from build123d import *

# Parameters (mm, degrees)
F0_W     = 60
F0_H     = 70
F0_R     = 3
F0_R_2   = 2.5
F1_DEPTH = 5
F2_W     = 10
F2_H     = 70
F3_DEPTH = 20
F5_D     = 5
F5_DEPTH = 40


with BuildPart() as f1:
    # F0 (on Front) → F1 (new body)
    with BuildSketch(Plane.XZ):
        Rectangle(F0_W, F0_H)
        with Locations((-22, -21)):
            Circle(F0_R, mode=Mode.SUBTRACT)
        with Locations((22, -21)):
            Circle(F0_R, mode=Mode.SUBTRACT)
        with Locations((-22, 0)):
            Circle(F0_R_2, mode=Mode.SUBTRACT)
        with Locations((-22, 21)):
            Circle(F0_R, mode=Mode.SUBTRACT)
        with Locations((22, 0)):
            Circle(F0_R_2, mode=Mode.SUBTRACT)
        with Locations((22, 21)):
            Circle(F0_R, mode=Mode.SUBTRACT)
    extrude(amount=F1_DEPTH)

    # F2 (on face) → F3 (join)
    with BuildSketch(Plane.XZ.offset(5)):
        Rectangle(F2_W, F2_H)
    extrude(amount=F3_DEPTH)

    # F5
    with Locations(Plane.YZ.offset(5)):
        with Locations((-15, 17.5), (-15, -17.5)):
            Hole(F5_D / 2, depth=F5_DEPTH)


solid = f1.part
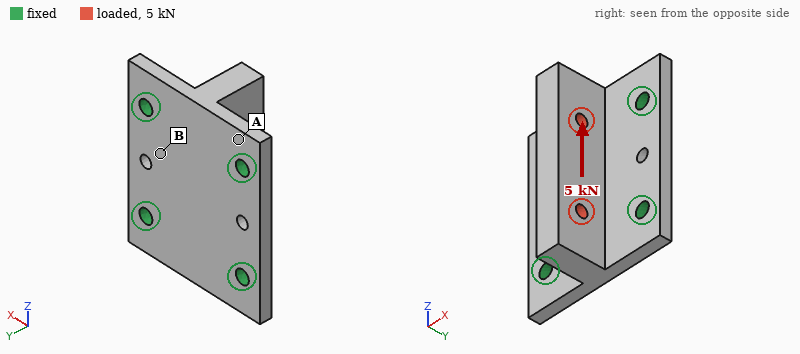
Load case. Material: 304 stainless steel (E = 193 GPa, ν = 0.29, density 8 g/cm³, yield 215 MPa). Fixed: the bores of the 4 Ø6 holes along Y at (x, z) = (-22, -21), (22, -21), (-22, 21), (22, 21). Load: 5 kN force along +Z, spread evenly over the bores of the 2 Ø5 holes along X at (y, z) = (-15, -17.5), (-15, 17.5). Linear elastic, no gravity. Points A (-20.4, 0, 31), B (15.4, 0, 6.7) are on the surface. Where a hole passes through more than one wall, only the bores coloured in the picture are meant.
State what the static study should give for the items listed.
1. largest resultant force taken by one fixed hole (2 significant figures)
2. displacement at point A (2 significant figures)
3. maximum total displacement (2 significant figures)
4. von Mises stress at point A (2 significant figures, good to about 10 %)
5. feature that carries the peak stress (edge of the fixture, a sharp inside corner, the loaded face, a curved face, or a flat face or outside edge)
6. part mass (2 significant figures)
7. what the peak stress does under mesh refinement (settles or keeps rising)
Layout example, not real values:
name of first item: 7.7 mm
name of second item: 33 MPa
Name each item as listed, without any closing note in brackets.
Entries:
largest resultant force taken by one fixed hole: 1.5 kN
displacement at point A: 2.8 µm
maximum total displacement: 18 µm
von Mises stress at point A: 26 MPa
feature that carries the peak stress: edge of the fixture
part mass: 270 g
what the peak stress does under mesh refinement: keeps rising
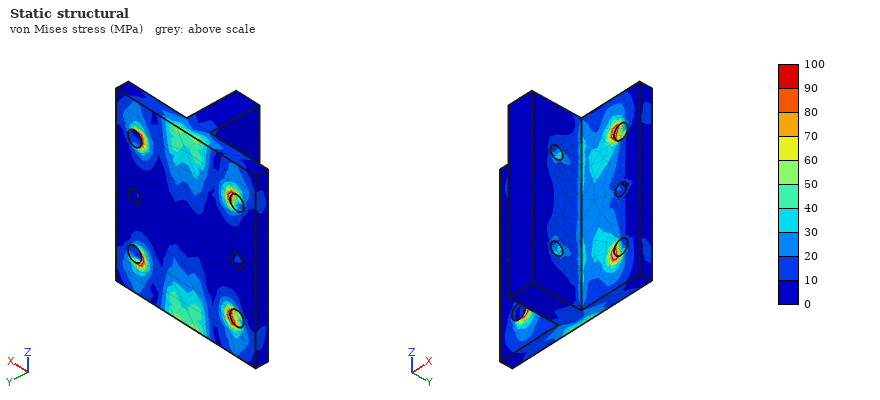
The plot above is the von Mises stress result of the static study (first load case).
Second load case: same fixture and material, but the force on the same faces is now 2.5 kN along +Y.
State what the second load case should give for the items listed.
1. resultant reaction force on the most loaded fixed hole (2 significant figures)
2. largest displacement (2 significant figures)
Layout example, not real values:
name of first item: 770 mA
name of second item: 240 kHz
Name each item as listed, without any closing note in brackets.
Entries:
resultant reaction force on the most loaded fixed hole: 640 N
largest displacement: 7.7 µm
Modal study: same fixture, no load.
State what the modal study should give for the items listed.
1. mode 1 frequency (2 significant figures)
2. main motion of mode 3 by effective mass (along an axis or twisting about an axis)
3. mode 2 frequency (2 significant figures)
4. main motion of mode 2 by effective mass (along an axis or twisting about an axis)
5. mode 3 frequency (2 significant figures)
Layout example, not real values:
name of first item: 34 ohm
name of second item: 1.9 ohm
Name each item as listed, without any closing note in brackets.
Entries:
mode 1 frequency: 6800 Hz
main motion of mode 3 by effective mass: along X
mode 2 frequency: 7100 Hz
main motion of mode 2 by effective mass: along Y
mode 3 frequency: 7800 Hz
